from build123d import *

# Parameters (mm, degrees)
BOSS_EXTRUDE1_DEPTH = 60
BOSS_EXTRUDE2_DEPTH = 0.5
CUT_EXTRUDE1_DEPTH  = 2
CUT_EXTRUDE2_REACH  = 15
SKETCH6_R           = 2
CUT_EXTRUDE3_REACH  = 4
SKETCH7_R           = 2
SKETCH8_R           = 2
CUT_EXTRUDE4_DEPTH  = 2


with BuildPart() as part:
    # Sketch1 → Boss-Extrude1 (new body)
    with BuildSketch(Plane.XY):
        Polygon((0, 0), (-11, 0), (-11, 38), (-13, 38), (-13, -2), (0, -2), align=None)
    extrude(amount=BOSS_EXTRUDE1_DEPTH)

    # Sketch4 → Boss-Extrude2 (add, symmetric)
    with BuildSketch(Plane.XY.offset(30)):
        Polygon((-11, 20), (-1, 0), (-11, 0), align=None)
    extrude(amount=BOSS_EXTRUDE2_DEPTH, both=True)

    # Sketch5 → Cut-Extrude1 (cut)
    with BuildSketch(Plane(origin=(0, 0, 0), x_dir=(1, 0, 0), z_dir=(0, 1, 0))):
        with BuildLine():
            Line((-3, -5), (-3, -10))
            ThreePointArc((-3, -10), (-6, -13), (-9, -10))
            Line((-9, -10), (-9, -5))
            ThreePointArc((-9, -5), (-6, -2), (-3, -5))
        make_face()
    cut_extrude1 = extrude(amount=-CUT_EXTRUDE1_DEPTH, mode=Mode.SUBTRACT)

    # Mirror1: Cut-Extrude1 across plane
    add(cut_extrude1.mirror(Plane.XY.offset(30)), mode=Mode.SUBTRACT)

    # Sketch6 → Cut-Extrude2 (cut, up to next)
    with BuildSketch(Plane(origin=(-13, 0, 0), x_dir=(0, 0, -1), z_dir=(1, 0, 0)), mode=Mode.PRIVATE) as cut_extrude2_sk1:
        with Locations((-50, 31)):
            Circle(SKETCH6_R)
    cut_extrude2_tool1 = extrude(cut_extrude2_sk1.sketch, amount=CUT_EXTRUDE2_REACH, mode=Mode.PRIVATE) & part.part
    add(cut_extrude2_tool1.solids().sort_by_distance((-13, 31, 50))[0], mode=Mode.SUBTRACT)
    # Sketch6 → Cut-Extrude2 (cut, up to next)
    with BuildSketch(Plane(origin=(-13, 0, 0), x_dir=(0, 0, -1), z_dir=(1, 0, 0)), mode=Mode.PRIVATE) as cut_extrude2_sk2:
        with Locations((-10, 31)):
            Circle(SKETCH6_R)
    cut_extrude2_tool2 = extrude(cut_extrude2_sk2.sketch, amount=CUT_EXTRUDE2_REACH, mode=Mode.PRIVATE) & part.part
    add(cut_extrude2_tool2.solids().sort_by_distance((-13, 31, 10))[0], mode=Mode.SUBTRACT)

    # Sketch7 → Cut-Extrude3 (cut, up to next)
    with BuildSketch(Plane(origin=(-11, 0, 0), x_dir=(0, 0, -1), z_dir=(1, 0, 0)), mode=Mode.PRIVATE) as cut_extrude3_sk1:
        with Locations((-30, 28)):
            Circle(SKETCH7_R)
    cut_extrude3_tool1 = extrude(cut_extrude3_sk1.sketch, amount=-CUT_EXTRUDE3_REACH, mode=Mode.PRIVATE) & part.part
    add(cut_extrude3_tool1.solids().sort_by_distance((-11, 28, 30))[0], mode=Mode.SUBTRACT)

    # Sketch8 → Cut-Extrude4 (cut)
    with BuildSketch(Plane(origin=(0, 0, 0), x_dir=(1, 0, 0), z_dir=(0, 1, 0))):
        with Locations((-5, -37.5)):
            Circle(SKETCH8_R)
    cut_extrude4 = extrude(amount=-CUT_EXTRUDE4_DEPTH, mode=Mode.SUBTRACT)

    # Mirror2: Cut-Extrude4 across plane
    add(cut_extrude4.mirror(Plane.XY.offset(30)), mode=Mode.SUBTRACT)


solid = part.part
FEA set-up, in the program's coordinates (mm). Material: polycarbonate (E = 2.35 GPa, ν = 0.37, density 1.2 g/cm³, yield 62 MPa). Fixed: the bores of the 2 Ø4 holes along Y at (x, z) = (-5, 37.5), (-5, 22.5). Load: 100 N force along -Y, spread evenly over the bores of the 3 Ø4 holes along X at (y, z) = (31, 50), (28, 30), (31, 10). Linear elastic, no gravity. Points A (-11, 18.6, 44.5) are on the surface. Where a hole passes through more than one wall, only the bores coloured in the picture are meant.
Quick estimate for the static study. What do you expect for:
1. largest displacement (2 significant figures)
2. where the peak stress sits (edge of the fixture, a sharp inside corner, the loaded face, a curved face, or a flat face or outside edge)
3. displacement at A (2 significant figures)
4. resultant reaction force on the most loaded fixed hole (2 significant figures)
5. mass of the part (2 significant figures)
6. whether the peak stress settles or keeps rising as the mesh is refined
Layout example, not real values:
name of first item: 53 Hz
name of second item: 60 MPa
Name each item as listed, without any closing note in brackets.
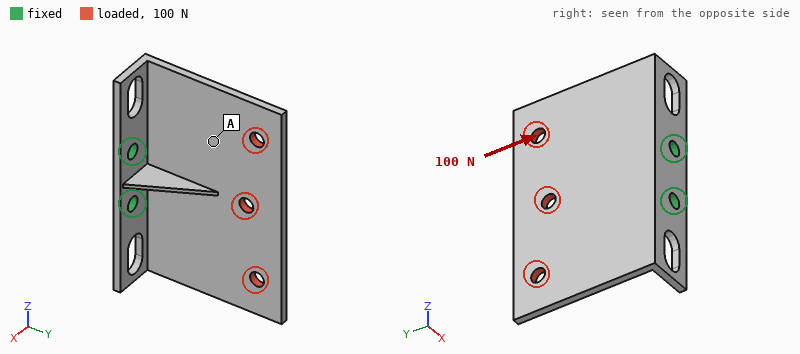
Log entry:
largest displacement: 0.83 mm
where the peak stress sits: edge of the fixture
displacement at A: 0.43 mm
resultant reaction force on the most loaded fixed hole: 50 N
mass of the part: 7.0 g
whether the peak stress settles or keeps rising as the mesh is refined: keeps rising
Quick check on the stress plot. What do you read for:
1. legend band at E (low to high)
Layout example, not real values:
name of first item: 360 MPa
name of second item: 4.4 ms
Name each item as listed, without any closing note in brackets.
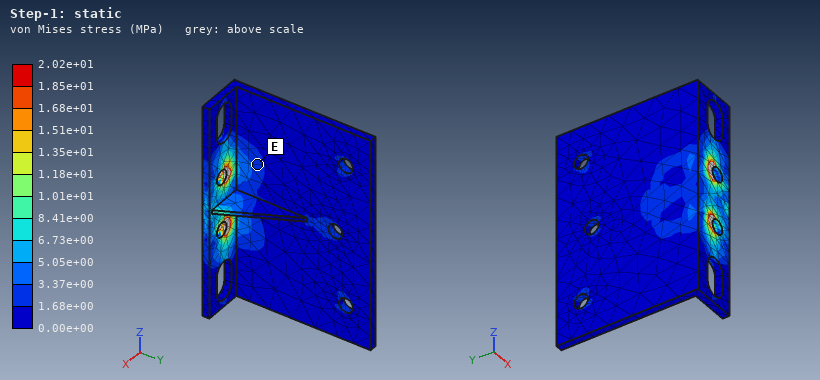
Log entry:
legend band at E: 1.68e+00 to 3.37e+00 MPa
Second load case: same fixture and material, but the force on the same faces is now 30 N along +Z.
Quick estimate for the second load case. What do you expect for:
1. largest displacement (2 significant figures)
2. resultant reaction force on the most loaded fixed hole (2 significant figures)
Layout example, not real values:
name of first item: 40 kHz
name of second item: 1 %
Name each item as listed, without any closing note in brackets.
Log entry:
largest displacement: 0.73 mm
resultant reaction force on the most loaded fixed hole: 54 N
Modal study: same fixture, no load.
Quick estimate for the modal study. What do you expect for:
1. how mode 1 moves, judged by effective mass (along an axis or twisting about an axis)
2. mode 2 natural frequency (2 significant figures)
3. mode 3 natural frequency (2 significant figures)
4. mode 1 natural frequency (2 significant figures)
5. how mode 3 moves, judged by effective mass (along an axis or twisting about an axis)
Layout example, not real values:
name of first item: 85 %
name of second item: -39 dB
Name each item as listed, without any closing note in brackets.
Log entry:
how mode 1 moves, judged by effective mass: along X
mode 2 natural frequency: 420 Hz
mode 3 natural frequency: 690 Hz
mode 1 natural frequency: 330 Hz
how mode 3 moves, judged by effective mass: along Z
